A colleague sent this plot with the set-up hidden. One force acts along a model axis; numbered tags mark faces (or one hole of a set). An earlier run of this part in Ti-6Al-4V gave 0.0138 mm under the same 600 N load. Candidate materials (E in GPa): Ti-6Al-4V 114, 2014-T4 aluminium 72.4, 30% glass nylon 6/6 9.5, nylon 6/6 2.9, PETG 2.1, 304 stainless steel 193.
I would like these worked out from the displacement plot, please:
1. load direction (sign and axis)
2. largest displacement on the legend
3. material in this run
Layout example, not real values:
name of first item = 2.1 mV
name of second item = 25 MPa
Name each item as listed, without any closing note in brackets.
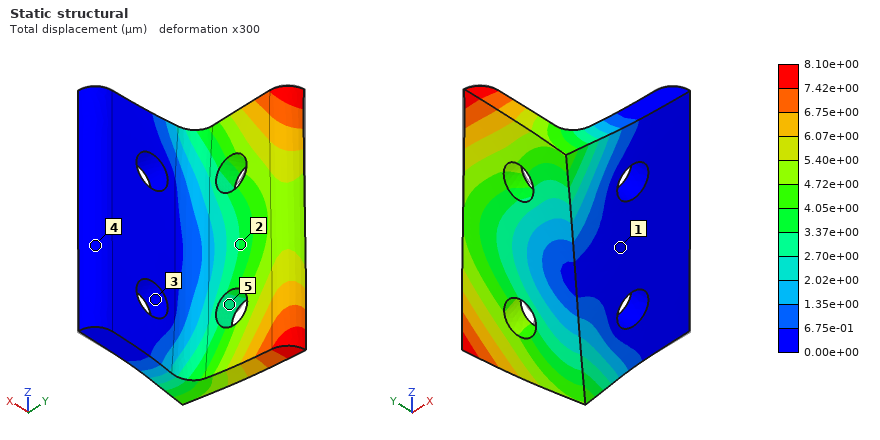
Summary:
load direction = -Z
largest displacement on the legend = 8.10e+00 µm
material in this run = 304 stainless steel
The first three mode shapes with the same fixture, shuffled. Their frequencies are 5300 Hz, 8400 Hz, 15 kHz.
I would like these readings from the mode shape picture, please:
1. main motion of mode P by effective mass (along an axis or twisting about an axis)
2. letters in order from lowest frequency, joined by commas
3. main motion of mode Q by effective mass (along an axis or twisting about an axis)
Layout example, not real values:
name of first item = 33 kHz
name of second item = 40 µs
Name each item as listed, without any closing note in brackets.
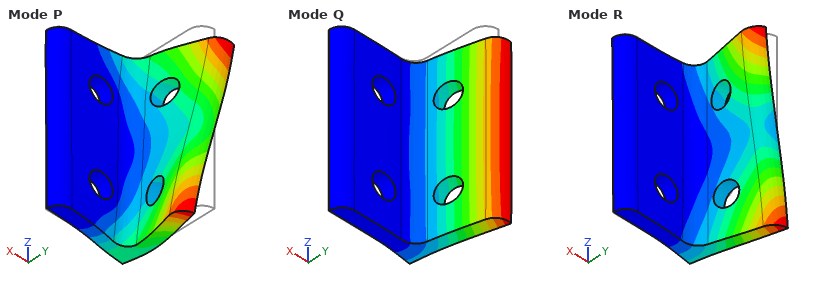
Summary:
main motion of mode P by effective mass = along Z
letters in order from lowest frequency, joined by commas = Q, R, P
main motion of mode Q by effective mass = along X
